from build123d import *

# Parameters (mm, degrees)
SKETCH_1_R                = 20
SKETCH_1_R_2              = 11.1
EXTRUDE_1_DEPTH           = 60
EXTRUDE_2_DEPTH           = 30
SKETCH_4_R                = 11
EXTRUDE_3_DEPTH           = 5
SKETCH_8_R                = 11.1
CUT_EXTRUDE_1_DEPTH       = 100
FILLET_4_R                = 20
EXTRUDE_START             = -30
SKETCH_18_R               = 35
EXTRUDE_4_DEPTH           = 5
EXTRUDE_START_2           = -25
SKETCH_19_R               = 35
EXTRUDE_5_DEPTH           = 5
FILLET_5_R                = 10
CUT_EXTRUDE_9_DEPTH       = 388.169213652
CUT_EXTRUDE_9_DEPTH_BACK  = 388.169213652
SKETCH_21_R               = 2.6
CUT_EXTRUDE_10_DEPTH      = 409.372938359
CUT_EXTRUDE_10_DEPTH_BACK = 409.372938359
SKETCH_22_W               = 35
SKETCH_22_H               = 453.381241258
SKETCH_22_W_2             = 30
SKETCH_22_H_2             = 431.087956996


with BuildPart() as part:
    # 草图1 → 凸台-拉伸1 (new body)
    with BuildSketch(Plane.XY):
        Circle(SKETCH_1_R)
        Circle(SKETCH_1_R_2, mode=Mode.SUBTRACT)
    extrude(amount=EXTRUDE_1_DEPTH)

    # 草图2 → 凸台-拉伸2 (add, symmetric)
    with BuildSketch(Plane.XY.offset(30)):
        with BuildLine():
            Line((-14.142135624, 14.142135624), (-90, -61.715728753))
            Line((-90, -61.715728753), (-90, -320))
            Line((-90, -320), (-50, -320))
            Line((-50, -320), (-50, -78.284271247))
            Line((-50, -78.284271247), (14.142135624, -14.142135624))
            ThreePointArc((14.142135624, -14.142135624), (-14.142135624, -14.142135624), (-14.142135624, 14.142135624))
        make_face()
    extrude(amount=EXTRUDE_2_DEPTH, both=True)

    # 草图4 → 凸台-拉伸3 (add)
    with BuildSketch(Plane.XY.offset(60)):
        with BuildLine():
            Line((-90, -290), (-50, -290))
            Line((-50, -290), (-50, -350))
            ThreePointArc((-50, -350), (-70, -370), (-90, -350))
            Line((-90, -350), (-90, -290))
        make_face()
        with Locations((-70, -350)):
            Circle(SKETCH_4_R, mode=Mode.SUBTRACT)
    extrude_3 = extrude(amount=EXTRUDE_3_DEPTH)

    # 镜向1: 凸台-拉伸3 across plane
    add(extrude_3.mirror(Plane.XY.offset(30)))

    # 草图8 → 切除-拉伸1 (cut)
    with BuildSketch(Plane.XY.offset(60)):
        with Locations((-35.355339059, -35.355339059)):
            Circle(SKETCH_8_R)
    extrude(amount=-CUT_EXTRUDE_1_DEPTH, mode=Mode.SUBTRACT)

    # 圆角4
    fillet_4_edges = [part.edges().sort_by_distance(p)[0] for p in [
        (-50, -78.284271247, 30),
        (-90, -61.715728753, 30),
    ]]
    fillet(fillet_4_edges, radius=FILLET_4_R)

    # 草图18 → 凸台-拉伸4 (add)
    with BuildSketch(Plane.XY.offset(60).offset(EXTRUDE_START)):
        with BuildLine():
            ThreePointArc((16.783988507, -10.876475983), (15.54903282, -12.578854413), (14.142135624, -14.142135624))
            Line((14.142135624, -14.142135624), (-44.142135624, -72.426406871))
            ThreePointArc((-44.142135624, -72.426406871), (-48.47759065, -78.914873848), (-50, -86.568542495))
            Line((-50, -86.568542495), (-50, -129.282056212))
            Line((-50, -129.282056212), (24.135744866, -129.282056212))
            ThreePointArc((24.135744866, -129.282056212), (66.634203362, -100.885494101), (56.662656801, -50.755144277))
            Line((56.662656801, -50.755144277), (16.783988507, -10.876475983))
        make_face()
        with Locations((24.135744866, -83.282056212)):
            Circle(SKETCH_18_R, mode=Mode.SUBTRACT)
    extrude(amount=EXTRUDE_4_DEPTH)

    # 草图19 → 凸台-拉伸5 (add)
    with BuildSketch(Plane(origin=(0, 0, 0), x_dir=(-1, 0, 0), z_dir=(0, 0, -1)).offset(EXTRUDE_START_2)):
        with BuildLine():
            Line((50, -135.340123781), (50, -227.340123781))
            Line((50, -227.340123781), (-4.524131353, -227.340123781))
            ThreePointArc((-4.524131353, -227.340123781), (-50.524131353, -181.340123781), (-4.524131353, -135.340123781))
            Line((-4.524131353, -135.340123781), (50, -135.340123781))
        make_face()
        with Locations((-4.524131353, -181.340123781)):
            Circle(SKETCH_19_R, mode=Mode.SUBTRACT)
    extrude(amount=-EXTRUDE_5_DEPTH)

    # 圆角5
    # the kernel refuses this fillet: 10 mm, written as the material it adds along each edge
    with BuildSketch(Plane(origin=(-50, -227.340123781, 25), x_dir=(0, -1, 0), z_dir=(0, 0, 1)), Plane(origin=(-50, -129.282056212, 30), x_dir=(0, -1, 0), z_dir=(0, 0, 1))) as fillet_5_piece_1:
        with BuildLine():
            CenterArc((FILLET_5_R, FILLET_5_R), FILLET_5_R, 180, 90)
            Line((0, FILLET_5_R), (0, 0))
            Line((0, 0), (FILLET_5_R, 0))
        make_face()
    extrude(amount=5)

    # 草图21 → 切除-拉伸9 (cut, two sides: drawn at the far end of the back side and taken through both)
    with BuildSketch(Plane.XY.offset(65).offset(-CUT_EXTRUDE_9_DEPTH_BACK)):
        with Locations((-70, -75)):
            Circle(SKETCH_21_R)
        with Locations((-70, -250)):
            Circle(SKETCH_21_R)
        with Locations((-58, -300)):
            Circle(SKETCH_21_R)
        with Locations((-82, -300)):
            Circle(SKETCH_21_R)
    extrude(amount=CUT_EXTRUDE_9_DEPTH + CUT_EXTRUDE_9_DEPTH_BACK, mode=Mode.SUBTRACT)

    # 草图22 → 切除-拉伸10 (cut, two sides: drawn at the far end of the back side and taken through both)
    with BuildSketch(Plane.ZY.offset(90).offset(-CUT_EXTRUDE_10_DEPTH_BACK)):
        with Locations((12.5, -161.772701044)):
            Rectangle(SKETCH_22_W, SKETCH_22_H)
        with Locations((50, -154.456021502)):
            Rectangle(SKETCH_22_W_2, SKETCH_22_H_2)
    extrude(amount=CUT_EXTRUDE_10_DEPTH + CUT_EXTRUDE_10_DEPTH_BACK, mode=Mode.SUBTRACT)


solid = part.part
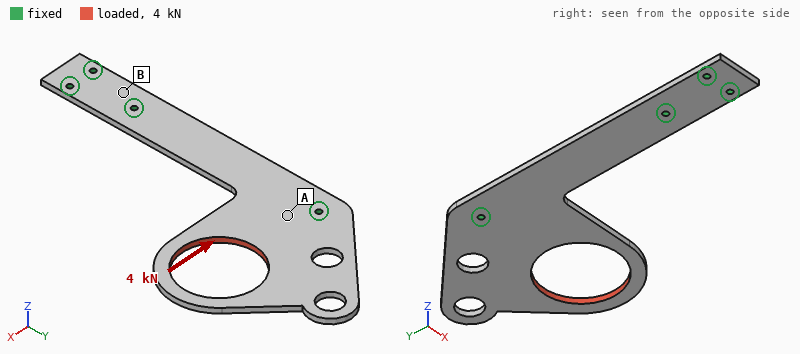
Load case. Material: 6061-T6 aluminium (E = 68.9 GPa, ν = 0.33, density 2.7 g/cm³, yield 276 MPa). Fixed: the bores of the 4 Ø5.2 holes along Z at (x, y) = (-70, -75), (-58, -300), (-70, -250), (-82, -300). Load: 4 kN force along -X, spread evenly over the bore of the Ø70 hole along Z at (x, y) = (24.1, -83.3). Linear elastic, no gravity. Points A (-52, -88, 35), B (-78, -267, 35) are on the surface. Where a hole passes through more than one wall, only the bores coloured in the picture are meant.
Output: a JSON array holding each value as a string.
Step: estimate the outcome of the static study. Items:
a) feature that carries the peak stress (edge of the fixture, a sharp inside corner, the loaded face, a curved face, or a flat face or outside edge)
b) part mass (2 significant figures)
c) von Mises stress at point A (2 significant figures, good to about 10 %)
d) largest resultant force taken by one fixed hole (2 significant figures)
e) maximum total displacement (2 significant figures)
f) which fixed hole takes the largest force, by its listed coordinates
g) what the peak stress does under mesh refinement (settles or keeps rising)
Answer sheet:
["edge of the fixture", "270 g", "13 MPa", "3.8 kN", "98 µm", "(-70, -75)", "keeps rising"]
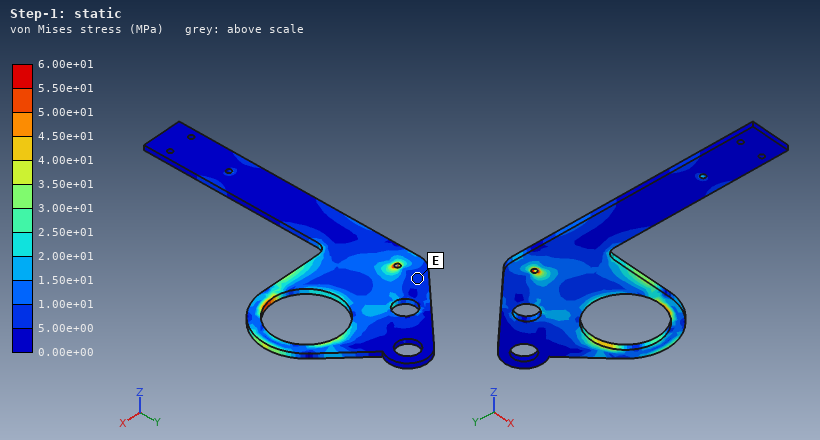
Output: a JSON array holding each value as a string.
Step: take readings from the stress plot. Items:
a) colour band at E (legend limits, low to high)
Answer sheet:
["5.00e+00 to 1.00e+01 MPa"]
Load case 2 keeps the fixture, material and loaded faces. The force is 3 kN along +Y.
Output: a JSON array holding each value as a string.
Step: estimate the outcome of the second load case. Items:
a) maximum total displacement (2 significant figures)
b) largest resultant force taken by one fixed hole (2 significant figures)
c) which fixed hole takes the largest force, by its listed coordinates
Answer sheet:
["0.60 mm", "3.1 kN", "(-70, -250)"]
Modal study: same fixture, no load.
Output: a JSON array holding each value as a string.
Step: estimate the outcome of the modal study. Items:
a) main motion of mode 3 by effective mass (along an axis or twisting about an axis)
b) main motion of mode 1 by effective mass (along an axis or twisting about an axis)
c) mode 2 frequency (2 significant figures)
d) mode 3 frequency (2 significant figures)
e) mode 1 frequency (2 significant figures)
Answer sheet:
["along Z", "along Z", "420 Hz", "830 Hz", "250 Hz"]
